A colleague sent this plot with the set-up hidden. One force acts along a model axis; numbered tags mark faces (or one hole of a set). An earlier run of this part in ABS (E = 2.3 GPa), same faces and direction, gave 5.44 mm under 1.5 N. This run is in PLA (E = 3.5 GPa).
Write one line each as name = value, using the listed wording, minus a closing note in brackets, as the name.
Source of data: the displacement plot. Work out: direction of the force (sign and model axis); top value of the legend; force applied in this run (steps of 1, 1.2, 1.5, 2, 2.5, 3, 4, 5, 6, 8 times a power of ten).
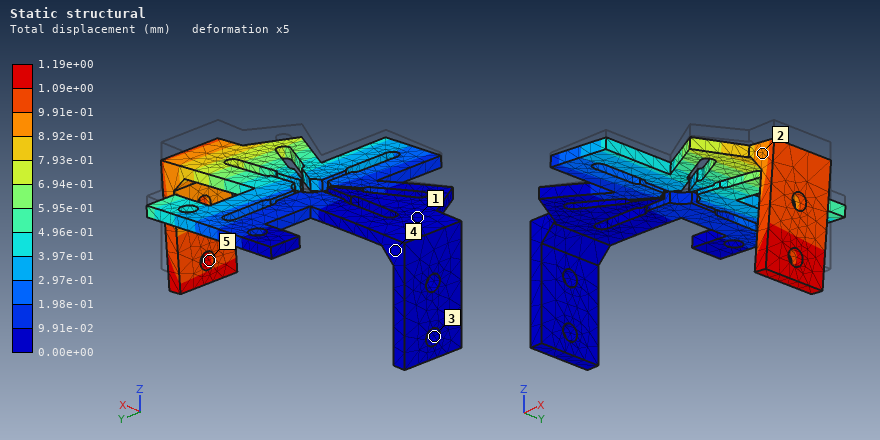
direction of the force = -Z
top value of the legend = 1.19e+00 mm
force applied in this run = 0.5 N
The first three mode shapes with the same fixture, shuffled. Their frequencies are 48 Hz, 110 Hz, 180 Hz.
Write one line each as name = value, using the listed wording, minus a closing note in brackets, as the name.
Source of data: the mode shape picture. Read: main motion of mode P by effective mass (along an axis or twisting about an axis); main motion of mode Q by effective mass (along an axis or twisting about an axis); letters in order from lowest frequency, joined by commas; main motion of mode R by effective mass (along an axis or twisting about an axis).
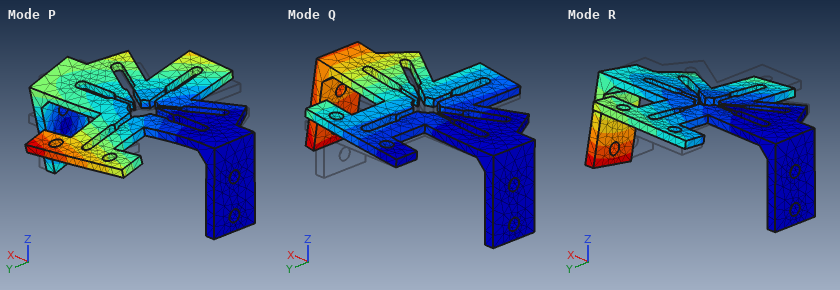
main motion of mode P by effective mass = along Y
main motion of mode Q by effective mass = along Z
letters in order from lowest frequency, joined by commas = Q, R, P
main motion of mode R by effective mass = along Y
